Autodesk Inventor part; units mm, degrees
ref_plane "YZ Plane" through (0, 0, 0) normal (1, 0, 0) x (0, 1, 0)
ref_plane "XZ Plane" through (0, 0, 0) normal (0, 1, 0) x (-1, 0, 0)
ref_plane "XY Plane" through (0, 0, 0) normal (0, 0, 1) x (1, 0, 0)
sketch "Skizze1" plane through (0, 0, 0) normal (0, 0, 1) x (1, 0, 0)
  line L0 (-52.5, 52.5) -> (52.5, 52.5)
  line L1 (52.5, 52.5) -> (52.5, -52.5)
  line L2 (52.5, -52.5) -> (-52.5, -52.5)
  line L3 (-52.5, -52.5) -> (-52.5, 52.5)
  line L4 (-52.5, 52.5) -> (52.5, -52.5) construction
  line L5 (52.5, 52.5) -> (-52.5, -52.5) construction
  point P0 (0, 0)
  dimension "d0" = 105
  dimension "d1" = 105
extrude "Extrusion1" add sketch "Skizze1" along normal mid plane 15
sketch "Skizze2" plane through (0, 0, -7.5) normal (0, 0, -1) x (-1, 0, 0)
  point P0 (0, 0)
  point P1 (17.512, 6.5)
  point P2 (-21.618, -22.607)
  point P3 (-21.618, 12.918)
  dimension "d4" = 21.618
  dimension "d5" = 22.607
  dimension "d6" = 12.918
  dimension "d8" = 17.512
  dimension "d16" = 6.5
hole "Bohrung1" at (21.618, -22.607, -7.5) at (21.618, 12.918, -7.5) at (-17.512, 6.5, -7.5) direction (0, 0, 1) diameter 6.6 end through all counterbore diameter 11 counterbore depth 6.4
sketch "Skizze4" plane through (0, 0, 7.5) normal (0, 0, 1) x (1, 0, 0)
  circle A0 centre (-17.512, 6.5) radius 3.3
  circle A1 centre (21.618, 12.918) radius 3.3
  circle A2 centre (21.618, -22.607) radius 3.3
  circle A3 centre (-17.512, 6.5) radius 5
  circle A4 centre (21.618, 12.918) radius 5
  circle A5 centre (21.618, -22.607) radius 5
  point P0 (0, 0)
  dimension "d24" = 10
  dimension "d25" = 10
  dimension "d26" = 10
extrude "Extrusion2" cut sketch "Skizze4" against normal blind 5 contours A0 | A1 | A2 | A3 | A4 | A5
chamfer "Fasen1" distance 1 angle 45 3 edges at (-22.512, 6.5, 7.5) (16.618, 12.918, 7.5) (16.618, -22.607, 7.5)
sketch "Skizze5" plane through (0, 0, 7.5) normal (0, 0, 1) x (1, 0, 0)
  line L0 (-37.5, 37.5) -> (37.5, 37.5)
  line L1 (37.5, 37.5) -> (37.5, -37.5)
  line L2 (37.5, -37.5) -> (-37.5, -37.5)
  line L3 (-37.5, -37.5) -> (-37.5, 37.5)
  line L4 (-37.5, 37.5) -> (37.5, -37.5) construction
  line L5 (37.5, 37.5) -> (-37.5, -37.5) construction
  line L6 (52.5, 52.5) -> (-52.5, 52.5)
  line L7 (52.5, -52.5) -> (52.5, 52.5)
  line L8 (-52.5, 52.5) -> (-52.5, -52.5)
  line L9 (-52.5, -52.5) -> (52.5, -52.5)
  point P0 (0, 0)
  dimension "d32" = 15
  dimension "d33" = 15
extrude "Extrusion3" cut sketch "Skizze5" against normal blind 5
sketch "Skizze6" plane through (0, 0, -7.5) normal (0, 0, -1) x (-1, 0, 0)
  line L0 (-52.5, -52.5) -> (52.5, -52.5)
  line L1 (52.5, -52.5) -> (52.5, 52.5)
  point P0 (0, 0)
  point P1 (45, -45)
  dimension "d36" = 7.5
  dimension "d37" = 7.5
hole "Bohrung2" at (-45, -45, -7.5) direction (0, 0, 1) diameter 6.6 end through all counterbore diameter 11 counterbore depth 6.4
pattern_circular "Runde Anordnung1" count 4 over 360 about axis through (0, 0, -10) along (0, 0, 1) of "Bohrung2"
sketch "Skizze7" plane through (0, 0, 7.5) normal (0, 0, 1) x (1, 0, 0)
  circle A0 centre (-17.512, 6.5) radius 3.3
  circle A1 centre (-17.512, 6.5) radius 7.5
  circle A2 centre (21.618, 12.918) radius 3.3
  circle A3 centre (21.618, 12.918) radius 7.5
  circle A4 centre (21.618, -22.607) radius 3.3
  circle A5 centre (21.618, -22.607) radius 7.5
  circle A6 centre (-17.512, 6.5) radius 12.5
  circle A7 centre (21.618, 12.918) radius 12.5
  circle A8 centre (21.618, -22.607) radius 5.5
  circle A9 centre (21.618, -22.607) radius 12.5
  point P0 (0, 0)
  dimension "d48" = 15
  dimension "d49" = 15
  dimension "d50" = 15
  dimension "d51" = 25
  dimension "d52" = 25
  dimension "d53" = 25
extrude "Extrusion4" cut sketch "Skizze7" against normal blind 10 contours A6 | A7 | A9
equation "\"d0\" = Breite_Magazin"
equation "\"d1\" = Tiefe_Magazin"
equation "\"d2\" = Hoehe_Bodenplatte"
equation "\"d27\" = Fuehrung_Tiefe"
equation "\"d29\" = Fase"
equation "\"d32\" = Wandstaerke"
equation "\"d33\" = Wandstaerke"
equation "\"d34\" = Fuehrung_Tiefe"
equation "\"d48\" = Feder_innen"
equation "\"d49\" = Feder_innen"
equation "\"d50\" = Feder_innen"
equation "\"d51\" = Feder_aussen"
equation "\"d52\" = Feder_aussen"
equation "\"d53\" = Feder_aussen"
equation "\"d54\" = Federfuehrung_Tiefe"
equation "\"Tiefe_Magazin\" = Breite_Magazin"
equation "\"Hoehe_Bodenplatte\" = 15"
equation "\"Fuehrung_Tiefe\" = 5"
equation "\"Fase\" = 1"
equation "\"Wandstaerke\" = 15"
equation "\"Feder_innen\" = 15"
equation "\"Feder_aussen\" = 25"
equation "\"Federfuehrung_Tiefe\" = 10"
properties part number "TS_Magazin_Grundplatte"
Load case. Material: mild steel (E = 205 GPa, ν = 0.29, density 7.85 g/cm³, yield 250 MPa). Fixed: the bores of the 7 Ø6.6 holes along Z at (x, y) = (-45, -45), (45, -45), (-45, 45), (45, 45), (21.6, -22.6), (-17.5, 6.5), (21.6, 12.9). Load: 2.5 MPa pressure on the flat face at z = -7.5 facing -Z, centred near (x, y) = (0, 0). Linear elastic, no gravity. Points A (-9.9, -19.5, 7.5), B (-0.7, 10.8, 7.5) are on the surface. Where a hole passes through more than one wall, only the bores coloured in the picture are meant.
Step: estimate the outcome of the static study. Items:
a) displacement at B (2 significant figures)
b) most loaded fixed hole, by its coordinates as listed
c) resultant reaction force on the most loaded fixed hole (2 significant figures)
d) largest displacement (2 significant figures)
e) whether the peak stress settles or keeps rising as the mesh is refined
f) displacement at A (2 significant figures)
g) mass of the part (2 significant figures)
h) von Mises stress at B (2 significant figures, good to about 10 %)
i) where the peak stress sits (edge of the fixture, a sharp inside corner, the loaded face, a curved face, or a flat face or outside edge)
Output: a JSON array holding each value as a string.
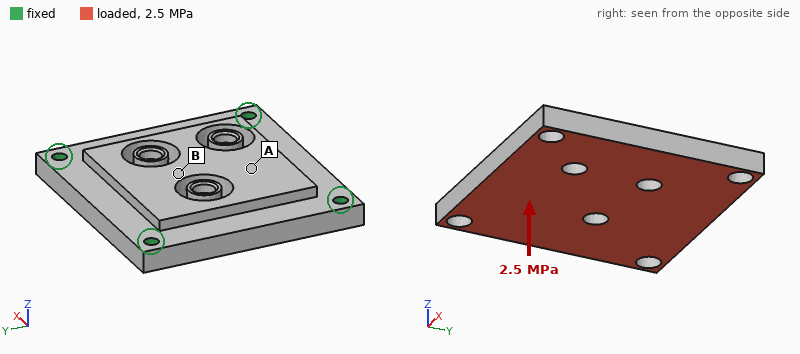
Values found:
["7.3 µm", "(-17.5, 6.5)", "6.1 kN", "19 µm", "keeps rising", "11 µm", "960 g", "25 MPa", "edge of the fixture"]
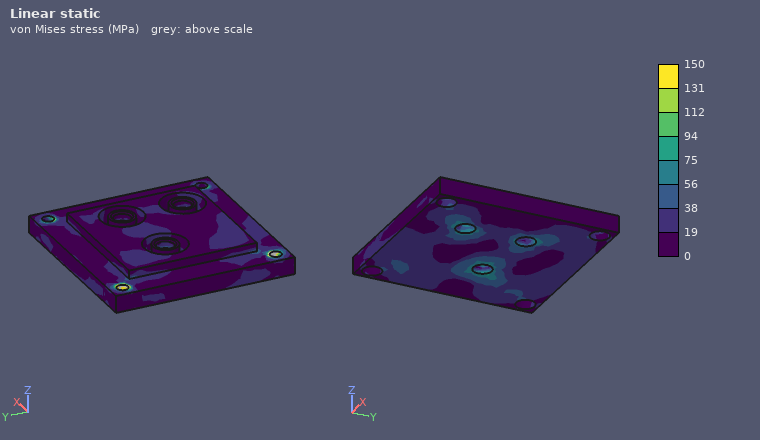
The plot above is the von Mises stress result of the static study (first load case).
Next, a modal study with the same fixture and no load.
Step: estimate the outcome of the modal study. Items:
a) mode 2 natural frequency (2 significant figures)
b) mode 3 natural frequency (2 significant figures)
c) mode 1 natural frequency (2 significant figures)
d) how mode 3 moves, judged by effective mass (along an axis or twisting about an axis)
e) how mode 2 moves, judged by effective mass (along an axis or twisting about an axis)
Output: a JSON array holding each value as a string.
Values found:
["7000 Hz", "7900 Hz", "6700 Hz", "along Z", "along Z"]
